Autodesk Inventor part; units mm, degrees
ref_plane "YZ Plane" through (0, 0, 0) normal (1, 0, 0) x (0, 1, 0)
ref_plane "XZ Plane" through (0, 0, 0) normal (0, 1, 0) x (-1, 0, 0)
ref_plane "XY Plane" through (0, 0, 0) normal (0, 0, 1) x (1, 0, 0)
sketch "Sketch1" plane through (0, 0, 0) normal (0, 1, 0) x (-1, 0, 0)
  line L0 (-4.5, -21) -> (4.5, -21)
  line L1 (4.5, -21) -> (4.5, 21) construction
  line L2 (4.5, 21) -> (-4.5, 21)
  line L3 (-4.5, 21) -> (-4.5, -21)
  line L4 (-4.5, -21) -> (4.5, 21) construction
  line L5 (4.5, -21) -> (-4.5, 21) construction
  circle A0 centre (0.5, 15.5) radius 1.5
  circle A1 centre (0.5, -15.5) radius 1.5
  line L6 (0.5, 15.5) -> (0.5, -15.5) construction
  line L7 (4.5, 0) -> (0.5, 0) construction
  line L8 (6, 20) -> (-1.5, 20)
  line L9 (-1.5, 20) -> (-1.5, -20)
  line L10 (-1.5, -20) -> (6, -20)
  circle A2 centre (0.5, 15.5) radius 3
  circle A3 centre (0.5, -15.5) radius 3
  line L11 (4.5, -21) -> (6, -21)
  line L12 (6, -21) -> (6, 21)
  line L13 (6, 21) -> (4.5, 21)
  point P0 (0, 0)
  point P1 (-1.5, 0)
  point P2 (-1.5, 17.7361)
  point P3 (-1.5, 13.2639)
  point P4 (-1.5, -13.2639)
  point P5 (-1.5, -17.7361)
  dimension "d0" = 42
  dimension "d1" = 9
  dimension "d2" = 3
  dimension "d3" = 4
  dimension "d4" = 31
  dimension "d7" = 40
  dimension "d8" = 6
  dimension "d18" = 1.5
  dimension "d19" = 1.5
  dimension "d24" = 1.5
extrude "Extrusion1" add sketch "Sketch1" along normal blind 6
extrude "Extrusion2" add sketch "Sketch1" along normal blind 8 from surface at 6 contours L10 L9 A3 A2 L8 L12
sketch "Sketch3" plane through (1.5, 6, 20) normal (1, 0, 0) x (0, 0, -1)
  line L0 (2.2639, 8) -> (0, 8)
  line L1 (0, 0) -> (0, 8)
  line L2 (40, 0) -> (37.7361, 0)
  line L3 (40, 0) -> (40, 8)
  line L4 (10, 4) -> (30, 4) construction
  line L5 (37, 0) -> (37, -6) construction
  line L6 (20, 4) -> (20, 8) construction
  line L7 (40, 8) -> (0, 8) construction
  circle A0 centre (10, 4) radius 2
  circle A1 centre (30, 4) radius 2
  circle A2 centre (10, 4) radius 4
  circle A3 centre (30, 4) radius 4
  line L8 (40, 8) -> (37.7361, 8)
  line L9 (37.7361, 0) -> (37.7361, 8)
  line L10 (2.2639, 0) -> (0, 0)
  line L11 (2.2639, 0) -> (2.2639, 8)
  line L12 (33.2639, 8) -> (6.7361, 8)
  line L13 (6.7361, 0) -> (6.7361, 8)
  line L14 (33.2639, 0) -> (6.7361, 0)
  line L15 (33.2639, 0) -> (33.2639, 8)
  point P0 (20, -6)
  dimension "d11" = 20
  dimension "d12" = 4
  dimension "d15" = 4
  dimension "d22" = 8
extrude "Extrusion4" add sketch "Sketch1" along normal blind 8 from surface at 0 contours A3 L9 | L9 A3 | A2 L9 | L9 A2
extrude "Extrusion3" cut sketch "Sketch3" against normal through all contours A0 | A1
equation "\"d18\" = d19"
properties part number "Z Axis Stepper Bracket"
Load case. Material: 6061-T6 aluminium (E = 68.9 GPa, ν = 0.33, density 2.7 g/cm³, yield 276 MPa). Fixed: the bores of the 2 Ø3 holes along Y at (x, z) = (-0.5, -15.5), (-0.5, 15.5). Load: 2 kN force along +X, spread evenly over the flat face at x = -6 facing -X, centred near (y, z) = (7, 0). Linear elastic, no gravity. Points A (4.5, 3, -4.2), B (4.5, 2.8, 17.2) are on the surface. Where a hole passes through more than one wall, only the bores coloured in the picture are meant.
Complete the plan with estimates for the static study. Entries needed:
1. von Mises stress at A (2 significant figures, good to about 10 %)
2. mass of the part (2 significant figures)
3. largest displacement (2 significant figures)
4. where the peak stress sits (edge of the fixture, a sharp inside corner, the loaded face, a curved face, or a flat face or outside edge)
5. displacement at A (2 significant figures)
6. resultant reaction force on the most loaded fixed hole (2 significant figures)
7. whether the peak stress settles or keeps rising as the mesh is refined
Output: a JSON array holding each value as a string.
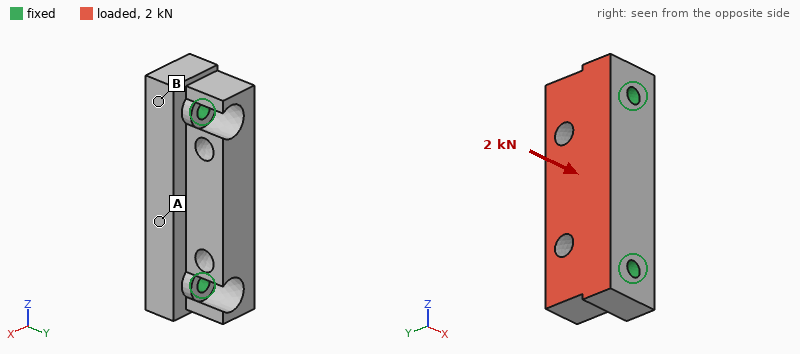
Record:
["16 MPa", "12 g", "14 µm", "edge of the fixture", "5.9 µm", "1.0 kN", "keeps rising"]
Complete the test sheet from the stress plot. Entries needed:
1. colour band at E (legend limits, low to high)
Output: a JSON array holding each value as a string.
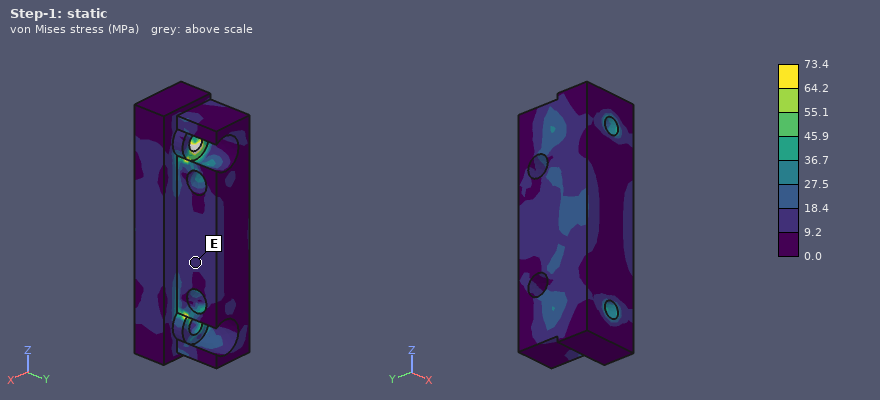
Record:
["9.2 to 18.4 MPa"]
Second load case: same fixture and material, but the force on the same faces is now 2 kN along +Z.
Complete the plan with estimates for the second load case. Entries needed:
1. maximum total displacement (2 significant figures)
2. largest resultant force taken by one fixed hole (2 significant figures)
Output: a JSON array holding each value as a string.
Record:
["4.4 µm", "1.1 kN"]
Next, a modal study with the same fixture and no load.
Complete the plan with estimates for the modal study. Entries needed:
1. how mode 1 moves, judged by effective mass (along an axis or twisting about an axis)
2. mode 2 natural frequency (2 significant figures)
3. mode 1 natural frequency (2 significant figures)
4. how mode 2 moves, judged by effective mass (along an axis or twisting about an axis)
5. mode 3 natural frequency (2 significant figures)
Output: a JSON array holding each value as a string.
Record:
["along X", "31 kHz", "22 kHz", "along Y", "33 kHz"]
